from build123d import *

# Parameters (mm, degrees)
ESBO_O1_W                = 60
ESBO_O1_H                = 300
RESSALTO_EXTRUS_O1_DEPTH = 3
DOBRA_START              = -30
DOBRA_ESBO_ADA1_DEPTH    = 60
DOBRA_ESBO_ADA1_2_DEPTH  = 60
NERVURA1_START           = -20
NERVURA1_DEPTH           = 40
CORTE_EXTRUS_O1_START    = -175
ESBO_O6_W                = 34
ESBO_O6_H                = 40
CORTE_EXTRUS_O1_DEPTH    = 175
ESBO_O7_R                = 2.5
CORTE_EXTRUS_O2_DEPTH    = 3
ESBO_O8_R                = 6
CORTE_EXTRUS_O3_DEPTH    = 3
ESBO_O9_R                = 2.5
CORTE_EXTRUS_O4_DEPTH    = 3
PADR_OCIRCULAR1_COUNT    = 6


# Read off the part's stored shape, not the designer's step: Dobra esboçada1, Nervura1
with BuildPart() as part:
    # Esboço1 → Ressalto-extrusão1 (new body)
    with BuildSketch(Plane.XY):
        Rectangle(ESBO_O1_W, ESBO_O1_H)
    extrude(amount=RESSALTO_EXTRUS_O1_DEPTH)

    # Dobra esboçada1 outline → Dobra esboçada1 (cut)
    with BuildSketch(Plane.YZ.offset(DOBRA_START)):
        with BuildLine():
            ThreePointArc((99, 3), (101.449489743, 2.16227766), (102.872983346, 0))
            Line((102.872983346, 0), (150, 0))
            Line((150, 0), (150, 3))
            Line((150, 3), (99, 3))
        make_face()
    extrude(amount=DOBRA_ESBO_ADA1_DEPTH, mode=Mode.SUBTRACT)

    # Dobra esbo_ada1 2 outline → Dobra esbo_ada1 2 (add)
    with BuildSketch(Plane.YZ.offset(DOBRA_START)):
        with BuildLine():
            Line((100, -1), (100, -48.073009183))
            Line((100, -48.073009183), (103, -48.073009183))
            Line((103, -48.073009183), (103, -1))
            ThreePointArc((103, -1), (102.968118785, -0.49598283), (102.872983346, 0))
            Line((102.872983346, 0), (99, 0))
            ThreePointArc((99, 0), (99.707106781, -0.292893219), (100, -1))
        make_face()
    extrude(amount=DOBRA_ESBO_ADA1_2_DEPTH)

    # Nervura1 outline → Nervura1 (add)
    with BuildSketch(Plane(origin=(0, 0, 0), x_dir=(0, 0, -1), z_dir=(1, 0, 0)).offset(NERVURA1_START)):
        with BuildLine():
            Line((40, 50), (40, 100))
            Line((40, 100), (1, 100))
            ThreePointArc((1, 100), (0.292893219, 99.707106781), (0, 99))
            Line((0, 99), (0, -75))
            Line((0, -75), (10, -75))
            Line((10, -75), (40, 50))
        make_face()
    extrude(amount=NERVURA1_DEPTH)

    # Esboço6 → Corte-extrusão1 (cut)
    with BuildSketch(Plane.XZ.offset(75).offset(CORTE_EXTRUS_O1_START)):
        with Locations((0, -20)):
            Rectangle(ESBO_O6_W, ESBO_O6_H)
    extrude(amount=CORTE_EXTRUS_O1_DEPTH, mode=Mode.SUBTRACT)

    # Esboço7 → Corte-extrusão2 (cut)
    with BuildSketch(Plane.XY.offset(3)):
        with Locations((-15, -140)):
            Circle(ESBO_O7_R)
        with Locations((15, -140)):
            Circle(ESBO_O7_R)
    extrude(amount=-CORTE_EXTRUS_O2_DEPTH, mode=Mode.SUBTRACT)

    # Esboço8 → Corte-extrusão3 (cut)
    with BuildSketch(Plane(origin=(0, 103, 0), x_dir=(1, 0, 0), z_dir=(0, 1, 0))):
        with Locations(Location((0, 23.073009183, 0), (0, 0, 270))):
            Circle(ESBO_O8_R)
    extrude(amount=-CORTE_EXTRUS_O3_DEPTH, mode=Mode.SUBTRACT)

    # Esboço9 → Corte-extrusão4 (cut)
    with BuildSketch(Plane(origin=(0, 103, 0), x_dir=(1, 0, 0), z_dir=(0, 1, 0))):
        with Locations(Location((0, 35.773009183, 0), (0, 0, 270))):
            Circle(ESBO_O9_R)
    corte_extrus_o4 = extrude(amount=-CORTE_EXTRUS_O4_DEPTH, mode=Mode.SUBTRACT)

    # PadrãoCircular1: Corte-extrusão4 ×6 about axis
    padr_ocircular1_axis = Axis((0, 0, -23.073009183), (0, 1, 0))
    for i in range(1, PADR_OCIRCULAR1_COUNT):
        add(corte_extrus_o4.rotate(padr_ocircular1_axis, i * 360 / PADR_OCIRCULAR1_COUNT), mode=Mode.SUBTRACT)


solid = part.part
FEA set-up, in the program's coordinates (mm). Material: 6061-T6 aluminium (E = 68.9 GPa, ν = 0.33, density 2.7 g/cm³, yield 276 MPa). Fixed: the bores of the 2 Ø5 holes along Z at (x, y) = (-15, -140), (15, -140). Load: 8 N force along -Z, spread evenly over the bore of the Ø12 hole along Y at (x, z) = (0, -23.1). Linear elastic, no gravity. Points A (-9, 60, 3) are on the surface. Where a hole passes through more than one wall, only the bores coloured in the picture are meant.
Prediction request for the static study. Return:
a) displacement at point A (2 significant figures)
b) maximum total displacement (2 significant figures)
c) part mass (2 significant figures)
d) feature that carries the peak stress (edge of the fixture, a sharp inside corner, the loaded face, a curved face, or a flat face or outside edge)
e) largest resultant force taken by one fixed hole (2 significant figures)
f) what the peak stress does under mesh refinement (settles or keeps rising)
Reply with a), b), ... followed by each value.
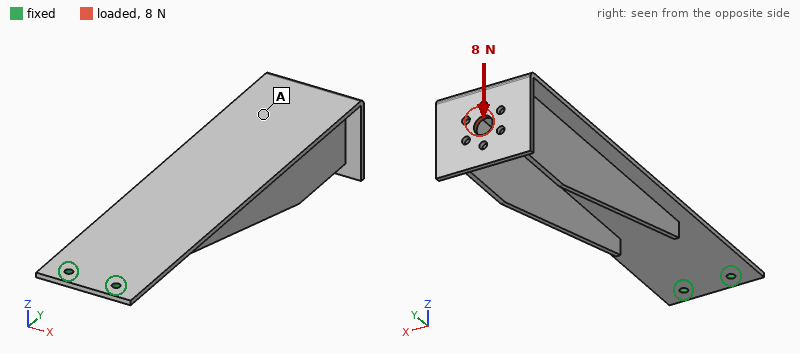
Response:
a) 2.0 mm
b) 2.6 mm
c) 230 g
d) edge of the fixture
e) 4.0 N
f) keeps rising
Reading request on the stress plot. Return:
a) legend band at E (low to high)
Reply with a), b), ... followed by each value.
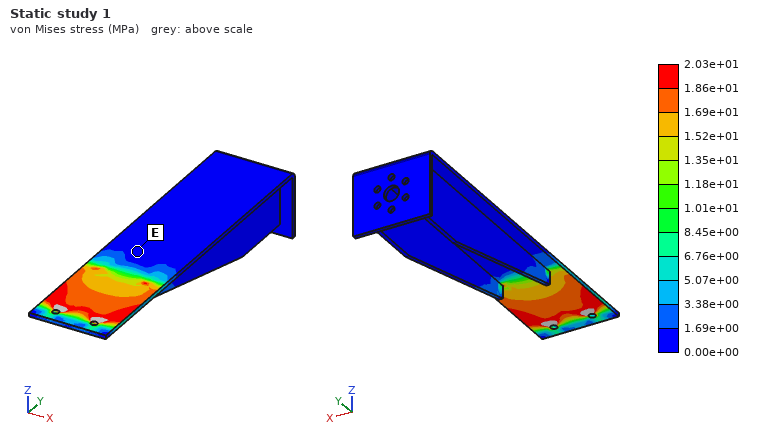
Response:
a) 0.00e+00 to 1.69e+00 MPa
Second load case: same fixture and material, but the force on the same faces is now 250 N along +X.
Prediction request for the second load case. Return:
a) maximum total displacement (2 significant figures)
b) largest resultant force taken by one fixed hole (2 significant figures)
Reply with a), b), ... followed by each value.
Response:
a) 3.1 mm
b) 1.8 kN
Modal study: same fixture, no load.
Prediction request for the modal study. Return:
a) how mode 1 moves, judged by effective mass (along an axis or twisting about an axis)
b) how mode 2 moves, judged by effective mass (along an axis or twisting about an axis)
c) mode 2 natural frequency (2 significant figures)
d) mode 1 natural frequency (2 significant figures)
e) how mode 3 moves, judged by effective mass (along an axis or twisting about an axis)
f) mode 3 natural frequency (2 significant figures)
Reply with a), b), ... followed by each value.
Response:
a) along Z
b) along X
c) 190 Hz
d) 29 Hz
e) along Z
f) 480 Hz
